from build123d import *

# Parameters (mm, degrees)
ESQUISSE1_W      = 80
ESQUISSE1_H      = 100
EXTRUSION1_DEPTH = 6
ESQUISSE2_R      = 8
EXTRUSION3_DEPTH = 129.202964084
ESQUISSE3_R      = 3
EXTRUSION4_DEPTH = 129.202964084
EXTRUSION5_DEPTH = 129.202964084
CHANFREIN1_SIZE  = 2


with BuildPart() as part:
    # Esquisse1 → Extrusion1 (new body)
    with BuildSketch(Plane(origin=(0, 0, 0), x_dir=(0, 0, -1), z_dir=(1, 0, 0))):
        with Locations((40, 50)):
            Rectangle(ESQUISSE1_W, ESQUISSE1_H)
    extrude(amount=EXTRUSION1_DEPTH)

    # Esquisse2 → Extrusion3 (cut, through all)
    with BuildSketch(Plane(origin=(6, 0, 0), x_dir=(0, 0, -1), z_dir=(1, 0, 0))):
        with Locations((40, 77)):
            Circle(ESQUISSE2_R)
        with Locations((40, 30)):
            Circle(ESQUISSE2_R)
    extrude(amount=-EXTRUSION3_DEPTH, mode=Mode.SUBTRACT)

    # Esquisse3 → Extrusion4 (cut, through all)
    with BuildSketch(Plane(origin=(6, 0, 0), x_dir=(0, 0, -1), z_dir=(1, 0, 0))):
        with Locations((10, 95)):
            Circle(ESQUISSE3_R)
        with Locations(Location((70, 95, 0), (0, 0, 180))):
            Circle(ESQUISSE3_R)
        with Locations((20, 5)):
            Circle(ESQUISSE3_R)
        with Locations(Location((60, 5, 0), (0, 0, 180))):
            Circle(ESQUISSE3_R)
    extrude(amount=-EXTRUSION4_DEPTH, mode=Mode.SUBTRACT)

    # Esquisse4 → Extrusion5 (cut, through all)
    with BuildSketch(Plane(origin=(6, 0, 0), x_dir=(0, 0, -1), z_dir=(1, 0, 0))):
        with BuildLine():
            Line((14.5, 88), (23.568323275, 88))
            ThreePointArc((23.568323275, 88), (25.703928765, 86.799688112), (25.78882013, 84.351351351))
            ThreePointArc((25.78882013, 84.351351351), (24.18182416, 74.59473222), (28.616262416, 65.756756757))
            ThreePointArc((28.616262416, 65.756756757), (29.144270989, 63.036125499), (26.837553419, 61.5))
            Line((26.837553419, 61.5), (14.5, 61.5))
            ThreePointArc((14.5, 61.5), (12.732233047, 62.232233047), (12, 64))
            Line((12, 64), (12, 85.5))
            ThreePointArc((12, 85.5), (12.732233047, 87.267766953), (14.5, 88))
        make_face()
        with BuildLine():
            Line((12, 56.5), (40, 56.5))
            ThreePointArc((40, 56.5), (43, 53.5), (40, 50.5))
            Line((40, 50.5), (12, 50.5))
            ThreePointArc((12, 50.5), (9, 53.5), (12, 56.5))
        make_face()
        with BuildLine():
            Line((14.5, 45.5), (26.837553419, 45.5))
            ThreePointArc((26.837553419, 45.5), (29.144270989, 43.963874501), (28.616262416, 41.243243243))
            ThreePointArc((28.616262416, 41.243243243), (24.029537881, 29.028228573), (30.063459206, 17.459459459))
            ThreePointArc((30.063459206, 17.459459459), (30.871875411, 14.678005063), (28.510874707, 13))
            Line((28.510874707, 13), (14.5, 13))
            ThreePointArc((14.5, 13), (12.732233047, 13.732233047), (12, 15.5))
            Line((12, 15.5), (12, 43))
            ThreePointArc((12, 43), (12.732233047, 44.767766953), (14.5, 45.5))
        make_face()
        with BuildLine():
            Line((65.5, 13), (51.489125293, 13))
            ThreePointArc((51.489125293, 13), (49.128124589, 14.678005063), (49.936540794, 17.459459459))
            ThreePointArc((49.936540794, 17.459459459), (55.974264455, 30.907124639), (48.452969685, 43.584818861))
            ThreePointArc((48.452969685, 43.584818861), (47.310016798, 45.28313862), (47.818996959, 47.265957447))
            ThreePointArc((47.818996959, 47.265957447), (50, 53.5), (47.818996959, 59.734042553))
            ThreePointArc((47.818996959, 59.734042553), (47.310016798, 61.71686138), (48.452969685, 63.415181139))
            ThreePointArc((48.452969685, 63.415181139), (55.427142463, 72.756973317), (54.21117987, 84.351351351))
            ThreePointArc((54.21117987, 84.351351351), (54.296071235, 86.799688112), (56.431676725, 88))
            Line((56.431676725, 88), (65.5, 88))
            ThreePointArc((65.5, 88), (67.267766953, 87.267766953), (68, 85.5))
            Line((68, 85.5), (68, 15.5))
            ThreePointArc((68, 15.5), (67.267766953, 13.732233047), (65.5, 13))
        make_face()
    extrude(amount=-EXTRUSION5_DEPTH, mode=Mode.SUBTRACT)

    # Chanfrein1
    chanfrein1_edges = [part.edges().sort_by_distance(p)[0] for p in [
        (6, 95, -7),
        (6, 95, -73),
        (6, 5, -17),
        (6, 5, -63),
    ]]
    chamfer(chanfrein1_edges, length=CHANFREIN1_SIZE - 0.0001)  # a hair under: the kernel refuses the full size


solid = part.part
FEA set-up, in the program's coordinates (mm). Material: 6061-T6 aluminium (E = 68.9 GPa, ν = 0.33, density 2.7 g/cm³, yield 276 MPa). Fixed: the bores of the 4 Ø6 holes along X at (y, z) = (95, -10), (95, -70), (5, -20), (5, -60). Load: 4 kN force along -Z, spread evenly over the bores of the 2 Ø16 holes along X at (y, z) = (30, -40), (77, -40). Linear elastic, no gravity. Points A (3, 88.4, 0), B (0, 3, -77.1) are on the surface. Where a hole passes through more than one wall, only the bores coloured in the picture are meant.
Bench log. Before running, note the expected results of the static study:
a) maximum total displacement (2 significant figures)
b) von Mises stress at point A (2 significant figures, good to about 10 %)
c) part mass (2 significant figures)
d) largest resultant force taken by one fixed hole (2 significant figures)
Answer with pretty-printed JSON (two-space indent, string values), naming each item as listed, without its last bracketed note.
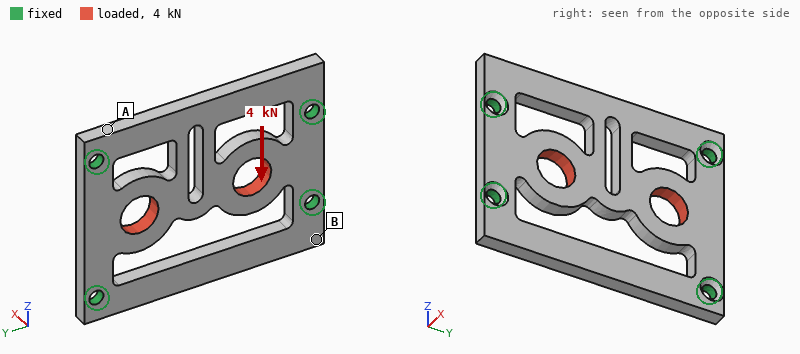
{
  "maximum total displacement": "49 µm",
  "von Mises stress at point A": "25 MPa",
  "part mass": "85 g",
  "largest resultant force taken by one fixed hole": "1.3 kN"
}
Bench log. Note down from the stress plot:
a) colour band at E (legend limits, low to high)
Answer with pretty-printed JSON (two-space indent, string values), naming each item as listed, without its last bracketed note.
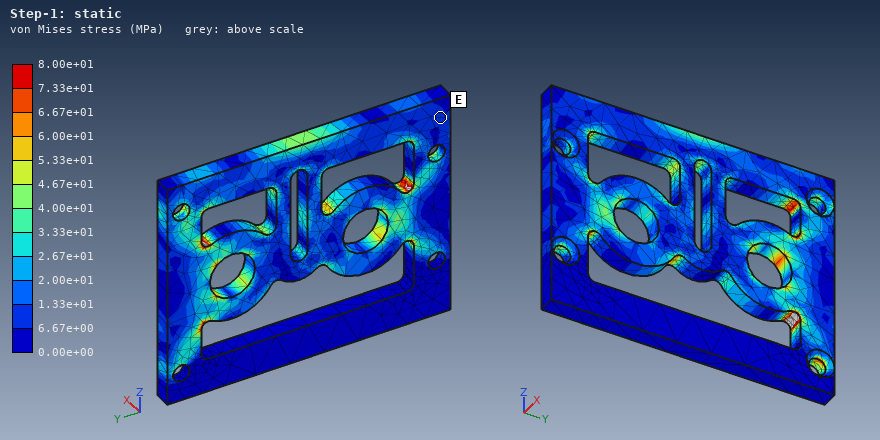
{
  "colour band at E": "6.67e+00 to 1.33e+01 MPa"
}
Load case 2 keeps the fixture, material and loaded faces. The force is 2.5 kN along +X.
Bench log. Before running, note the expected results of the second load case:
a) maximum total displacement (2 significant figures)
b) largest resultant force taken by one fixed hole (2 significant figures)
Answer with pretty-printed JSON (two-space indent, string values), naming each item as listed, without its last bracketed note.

{
  "maximum total displacement": "0.36 mm",
  "largest resultant force taken by one fixed hole": "720 N"
}
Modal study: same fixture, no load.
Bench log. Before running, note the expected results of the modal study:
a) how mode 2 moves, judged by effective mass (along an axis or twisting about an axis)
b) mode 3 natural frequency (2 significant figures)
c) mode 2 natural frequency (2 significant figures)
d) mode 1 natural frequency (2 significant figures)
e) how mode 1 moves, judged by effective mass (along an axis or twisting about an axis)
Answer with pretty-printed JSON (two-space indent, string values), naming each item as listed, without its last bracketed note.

{
  "how mode 2 moves, judged by effective mass": "along X",
  "mode 3 natural frequency": "3900 Hz",
  "mode 2 natural frequency": "3300 Hz",
  "mode 1 natural frequency": "2700 Hz",
  "how mode 1 moves, judged by effective mass": "along X"
}
